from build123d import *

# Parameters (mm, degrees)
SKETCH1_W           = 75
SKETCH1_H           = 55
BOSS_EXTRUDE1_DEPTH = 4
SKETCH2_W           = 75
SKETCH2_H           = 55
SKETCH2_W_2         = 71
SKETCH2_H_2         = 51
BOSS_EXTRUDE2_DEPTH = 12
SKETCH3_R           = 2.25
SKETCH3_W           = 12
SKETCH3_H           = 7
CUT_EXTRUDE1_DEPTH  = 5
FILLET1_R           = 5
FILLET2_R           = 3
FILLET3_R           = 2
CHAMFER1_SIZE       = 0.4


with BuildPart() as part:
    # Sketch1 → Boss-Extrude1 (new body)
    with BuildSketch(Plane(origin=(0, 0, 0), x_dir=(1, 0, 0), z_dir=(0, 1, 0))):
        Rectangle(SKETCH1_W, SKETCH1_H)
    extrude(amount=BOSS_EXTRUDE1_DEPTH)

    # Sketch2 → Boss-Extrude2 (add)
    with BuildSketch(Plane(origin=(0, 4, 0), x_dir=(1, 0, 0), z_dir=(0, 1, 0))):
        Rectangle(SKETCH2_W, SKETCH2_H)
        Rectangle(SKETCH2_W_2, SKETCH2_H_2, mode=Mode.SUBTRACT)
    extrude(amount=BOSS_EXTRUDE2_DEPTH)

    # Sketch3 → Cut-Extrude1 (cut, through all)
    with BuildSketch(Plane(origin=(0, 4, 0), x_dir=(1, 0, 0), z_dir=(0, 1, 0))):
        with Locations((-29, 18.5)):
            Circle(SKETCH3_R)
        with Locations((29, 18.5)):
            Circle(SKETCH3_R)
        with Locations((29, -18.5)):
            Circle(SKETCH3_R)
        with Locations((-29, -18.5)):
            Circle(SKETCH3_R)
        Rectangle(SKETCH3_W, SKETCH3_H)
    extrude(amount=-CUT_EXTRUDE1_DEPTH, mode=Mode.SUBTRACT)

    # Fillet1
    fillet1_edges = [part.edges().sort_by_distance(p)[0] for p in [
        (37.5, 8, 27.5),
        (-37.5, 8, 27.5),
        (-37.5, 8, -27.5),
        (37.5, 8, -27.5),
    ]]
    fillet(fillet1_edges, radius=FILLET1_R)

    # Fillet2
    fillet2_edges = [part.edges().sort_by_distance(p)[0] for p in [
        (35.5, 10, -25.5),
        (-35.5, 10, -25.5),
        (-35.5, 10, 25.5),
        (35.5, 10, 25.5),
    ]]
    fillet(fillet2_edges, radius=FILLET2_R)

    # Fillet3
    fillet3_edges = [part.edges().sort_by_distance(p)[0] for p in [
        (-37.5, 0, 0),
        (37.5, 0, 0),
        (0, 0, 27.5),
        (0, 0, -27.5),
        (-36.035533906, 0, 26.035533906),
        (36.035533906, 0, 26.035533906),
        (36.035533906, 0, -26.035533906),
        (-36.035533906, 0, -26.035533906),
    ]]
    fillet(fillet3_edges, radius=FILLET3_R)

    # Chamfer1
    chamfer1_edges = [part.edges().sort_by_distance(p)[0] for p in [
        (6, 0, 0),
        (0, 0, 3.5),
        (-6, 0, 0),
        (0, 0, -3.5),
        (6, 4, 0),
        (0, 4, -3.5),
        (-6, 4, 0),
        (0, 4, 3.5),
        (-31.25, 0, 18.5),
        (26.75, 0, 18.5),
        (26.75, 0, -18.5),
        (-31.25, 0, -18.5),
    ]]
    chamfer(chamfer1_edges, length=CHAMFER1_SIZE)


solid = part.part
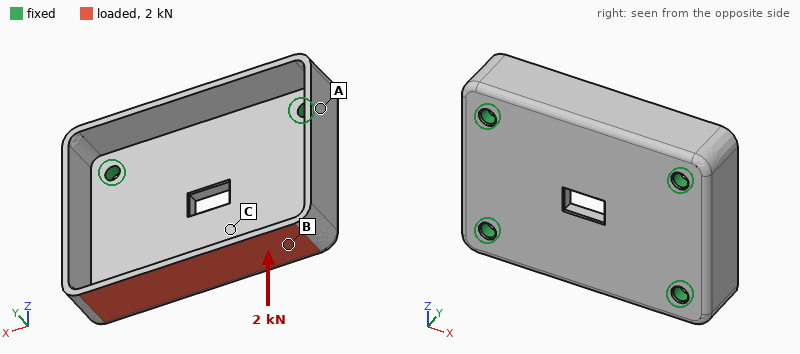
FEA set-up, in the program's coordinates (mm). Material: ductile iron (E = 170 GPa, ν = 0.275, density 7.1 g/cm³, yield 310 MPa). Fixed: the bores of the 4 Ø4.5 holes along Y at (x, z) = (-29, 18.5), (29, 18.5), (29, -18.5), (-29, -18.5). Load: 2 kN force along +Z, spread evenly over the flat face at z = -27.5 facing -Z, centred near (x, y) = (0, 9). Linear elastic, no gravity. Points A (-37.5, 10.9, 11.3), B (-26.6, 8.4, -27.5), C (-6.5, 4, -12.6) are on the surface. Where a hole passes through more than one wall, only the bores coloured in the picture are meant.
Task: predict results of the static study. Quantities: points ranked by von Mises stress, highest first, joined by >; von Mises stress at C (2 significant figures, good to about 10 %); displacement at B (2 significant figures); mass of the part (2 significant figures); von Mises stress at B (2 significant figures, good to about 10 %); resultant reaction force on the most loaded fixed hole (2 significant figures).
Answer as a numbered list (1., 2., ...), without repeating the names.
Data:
1. B > C > A
2. 33 MPa
3. 18 µm
4. 150 g
5. 96 MPa
6. 610 N
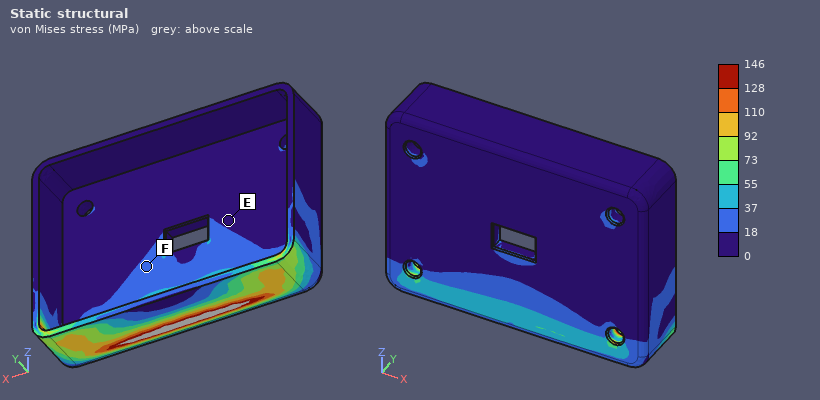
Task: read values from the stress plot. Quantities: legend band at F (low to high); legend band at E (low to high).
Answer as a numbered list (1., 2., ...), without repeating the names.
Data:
1. 18 to 37 MPa
2. 0 to 18 MPa
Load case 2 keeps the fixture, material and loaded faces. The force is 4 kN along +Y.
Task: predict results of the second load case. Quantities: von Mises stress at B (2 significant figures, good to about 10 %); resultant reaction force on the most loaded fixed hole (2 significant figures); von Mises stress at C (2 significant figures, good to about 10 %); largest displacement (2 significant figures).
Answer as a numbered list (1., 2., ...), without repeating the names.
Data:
1. 120 MPa
2. 2.5 kN
3. 50 MPa
4. 94 µm
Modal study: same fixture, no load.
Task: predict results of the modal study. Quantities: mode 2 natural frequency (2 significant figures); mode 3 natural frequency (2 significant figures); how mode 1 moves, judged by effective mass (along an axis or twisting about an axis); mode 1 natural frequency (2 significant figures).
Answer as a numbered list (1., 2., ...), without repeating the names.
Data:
1. 8200 Hz
2. 8300 Hz
3. along Y
4. 6200 Hz
